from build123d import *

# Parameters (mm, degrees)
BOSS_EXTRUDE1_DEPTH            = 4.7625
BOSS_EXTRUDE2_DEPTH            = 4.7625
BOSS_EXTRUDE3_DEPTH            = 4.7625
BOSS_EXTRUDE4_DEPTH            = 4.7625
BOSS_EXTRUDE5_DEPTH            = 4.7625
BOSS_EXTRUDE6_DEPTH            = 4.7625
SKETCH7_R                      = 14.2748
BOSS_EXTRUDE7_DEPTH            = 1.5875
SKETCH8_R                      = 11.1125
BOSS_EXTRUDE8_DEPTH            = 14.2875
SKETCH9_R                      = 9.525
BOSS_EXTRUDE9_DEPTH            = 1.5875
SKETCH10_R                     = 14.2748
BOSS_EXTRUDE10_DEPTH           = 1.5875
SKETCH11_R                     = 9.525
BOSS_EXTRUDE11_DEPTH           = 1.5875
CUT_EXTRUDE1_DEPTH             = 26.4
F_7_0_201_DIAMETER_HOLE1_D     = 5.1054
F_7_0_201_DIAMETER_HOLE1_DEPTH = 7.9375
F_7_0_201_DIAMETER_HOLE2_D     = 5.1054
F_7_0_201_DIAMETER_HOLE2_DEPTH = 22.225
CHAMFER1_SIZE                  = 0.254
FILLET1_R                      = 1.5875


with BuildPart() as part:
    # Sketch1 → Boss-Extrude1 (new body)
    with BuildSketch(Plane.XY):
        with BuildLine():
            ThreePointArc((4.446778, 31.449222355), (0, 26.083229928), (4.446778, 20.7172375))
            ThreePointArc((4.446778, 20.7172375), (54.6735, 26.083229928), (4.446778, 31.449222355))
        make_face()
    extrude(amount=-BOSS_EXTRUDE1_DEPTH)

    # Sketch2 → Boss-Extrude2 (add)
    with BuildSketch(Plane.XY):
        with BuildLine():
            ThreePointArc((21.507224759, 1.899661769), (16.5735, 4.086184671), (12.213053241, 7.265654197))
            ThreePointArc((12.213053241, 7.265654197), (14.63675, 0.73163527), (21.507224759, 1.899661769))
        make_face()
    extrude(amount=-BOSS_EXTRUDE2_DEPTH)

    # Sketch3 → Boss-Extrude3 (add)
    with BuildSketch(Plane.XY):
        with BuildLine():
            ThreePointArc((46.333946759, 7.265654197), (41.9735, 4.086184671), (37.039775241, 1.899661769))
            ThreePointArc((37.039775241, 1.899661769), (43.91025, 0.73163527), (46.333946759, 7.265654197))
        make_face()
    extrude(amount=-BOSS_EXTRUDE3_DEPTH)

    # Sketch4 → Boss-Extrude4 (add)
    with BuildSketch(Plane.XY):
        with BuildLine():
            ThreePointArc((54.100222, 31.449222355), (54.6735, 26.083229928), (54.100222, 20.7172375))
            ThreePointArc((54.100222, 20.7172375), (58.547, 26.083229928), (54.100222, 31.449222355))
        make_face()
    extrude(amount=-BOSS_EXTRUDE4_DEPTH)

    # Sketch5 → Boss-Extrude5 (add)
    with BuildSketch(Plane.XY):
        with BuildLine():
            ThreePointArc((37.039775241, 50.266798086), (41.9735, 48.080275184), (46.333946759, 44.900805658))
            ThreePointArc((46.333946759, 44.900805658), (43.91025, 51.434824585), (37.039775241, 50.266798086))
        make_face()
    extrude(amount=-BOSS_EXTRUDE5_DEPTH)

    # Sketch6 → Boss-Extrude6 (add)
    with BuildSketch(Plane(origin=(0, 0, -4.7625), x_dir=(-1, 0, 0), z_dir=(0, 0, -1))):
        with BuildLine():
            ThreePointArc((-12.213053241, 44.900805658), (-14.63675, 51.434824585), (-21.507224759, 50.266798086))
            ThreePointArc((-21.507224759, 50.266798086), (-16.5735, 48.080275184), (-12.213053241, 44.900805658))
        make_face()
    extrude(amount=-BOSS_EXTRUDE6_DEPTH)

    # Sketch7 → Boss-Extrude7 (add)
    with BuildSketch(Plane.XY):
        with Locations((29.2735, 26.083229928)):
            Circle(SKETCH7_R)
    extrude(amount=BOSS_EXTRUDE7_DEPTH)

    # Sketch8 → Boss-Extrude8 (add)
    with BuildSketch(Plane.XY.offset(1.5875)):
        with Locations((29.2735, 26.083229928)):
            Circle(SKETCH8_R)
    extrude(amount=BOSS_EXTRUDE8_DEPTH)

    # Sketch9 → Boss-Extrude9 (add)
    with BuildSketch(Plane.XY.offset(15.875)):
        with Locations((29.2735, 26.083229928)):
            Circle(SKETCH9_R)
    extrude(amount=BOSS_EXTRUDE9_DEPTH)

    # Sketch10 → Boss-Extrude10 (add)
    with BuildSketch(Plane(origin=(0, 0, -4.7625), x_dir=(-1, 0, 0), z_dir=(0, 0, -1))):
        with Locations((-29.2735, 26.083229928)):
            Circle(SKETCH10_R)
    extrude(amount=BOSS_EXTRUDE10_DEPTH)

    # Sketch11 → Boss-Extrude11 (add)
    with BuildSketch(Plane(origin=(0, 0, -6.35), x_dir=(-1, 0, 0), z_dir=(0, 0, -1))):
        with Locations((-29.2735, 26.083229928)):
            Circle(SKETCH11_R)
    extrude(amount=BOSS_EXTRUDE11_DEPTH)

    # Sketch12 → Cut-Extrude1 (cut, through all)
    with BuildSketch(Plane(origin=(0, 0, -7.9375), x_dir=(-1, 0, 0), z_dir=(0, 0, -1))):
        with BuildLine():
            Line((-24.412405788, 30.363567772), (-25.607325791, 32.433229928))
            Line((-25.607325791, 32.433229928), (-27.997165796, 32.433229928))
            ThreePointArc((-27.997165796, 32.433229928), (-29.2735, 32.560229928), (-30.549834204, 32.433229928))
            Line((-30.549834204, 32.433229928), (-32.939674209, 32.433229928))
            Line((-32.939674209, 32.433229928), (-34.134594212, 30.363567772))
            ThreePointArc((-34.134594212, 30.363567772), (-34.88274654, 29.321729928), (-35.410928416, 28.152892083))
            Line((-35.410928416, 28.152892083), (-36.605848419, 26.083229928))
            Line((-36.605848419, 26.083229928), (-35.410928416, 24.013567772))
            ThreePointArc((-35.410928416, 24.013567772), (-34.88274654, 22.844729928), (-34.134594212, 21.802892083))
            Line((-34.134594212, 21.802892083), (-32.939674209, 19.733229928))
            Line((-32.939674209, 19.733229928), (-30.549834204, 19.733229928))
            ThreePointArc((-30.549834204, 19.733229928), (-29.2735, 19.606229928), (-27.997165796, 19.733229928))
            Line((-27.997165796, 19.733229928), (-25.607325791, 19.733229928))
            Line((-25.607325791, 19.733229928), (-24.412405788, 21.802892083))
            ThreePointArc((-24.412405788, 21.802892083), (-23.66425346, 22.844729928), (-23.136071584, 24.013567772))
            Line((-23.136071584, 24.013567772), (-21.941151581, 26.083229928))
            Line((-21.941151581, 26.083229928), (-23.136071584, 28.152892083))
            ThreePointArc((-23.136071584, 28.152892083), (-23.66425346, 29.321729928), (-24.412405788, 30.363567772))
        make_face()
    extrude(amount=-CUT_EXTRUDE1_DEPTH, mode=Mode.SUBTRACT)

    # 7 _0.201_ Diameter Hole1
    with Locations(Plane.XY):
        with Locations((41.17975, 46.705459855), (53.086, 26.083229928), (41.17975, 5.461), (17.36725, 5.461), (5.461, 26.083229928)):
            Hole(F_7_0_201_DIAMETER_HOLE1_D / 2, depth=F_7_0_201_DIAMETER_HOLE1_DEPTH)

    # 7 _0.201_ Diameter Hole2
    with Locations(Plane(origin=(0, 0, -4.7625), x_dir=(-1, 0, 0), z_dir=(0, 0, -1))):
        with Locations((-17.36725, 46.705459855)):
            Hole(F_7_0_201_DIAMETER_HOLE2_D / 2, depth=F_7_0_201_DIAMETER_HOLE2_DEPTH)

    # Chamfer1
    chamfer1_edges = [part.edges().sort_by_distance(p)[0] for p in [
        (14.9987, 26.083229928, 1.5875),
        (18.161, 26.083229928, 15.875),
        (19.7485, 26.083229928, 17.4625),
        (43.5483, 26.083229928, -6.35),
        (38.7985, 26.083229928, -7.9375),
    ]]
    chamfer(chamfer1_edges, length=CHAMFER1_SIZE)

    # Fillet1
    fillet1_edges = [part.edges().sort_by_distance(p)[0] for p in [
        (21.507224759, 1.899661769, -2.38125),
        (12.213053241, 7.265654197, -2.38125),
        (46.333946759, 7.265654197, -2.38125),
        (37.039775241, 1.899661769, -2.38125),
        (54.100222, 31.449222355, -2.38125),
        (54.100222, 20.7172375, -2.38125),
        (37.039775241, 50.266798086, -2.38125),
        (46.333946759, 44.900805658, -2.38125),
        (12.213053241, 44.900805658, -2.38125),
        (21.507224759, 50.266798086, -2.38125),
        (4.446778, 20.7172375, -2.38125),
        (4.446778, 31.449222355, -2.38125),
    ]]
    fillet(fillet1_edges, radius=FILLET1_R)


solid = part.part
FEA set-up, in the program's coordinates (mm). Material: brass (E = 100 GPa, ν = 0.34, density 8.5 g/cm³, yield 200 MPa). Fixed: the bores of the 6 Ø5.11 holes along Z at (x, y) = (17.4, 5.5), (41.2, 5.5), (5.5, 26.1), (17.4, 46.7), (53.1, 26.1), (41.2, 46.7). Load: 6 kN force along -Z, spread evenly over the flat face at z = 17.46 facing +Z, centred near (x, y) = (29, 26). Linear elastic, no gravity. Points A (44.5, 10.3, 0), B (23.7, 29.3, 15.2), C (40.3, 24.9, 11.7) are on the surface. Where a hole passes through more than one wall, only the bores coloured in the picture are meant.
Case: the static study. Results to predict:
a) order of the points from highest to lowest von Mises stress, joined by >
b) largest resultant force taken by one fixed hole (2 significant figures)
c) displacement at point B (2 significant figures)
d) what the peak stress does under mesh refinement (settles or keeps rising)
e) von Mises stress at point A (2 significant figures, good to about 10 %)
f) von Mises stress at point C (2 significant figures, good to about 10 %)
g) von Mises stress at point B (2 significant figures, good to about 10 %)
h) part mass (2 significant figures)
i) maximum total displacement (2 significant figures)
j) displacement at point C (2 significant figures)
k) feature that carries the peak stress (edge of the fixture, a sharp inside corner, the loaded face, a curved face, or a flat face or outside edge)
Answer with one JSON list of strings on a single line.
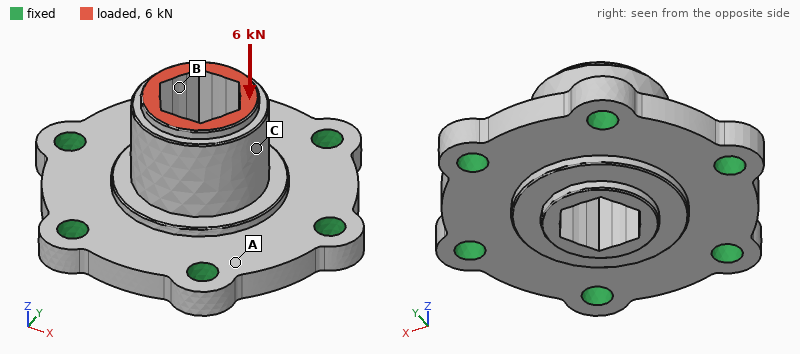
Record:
["B > A > C", "1.0 kN", "20 µm", "keeps rising", "27 MPa", "13 MPa", "48 MPa", "130 g", "21 µm", "18 µm", "edge of the fixture"]
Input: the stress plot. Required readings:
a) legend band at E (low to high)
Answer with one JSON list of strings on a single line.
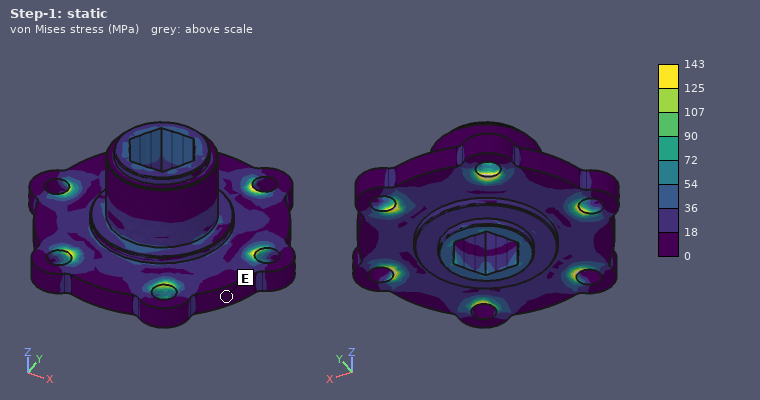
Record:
["0 to 18 MPa"]
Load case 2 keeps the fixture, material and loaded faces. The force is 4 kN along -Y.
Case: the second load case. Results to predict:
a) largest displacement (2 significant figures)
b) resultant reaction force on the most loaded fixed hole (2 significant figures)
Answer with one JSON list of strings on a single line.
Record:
["51 µm", "1.5 kN"]
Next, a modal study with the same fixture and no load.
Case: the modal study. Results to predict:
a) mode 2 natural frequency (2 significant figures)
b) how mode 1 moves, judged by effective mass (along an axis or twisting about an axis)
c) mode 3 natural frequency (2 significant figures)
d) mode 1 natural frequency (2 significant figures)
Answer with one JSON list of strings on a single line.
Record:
["12 kHz", "along Z", "13 kHz", "12 kHz"]
